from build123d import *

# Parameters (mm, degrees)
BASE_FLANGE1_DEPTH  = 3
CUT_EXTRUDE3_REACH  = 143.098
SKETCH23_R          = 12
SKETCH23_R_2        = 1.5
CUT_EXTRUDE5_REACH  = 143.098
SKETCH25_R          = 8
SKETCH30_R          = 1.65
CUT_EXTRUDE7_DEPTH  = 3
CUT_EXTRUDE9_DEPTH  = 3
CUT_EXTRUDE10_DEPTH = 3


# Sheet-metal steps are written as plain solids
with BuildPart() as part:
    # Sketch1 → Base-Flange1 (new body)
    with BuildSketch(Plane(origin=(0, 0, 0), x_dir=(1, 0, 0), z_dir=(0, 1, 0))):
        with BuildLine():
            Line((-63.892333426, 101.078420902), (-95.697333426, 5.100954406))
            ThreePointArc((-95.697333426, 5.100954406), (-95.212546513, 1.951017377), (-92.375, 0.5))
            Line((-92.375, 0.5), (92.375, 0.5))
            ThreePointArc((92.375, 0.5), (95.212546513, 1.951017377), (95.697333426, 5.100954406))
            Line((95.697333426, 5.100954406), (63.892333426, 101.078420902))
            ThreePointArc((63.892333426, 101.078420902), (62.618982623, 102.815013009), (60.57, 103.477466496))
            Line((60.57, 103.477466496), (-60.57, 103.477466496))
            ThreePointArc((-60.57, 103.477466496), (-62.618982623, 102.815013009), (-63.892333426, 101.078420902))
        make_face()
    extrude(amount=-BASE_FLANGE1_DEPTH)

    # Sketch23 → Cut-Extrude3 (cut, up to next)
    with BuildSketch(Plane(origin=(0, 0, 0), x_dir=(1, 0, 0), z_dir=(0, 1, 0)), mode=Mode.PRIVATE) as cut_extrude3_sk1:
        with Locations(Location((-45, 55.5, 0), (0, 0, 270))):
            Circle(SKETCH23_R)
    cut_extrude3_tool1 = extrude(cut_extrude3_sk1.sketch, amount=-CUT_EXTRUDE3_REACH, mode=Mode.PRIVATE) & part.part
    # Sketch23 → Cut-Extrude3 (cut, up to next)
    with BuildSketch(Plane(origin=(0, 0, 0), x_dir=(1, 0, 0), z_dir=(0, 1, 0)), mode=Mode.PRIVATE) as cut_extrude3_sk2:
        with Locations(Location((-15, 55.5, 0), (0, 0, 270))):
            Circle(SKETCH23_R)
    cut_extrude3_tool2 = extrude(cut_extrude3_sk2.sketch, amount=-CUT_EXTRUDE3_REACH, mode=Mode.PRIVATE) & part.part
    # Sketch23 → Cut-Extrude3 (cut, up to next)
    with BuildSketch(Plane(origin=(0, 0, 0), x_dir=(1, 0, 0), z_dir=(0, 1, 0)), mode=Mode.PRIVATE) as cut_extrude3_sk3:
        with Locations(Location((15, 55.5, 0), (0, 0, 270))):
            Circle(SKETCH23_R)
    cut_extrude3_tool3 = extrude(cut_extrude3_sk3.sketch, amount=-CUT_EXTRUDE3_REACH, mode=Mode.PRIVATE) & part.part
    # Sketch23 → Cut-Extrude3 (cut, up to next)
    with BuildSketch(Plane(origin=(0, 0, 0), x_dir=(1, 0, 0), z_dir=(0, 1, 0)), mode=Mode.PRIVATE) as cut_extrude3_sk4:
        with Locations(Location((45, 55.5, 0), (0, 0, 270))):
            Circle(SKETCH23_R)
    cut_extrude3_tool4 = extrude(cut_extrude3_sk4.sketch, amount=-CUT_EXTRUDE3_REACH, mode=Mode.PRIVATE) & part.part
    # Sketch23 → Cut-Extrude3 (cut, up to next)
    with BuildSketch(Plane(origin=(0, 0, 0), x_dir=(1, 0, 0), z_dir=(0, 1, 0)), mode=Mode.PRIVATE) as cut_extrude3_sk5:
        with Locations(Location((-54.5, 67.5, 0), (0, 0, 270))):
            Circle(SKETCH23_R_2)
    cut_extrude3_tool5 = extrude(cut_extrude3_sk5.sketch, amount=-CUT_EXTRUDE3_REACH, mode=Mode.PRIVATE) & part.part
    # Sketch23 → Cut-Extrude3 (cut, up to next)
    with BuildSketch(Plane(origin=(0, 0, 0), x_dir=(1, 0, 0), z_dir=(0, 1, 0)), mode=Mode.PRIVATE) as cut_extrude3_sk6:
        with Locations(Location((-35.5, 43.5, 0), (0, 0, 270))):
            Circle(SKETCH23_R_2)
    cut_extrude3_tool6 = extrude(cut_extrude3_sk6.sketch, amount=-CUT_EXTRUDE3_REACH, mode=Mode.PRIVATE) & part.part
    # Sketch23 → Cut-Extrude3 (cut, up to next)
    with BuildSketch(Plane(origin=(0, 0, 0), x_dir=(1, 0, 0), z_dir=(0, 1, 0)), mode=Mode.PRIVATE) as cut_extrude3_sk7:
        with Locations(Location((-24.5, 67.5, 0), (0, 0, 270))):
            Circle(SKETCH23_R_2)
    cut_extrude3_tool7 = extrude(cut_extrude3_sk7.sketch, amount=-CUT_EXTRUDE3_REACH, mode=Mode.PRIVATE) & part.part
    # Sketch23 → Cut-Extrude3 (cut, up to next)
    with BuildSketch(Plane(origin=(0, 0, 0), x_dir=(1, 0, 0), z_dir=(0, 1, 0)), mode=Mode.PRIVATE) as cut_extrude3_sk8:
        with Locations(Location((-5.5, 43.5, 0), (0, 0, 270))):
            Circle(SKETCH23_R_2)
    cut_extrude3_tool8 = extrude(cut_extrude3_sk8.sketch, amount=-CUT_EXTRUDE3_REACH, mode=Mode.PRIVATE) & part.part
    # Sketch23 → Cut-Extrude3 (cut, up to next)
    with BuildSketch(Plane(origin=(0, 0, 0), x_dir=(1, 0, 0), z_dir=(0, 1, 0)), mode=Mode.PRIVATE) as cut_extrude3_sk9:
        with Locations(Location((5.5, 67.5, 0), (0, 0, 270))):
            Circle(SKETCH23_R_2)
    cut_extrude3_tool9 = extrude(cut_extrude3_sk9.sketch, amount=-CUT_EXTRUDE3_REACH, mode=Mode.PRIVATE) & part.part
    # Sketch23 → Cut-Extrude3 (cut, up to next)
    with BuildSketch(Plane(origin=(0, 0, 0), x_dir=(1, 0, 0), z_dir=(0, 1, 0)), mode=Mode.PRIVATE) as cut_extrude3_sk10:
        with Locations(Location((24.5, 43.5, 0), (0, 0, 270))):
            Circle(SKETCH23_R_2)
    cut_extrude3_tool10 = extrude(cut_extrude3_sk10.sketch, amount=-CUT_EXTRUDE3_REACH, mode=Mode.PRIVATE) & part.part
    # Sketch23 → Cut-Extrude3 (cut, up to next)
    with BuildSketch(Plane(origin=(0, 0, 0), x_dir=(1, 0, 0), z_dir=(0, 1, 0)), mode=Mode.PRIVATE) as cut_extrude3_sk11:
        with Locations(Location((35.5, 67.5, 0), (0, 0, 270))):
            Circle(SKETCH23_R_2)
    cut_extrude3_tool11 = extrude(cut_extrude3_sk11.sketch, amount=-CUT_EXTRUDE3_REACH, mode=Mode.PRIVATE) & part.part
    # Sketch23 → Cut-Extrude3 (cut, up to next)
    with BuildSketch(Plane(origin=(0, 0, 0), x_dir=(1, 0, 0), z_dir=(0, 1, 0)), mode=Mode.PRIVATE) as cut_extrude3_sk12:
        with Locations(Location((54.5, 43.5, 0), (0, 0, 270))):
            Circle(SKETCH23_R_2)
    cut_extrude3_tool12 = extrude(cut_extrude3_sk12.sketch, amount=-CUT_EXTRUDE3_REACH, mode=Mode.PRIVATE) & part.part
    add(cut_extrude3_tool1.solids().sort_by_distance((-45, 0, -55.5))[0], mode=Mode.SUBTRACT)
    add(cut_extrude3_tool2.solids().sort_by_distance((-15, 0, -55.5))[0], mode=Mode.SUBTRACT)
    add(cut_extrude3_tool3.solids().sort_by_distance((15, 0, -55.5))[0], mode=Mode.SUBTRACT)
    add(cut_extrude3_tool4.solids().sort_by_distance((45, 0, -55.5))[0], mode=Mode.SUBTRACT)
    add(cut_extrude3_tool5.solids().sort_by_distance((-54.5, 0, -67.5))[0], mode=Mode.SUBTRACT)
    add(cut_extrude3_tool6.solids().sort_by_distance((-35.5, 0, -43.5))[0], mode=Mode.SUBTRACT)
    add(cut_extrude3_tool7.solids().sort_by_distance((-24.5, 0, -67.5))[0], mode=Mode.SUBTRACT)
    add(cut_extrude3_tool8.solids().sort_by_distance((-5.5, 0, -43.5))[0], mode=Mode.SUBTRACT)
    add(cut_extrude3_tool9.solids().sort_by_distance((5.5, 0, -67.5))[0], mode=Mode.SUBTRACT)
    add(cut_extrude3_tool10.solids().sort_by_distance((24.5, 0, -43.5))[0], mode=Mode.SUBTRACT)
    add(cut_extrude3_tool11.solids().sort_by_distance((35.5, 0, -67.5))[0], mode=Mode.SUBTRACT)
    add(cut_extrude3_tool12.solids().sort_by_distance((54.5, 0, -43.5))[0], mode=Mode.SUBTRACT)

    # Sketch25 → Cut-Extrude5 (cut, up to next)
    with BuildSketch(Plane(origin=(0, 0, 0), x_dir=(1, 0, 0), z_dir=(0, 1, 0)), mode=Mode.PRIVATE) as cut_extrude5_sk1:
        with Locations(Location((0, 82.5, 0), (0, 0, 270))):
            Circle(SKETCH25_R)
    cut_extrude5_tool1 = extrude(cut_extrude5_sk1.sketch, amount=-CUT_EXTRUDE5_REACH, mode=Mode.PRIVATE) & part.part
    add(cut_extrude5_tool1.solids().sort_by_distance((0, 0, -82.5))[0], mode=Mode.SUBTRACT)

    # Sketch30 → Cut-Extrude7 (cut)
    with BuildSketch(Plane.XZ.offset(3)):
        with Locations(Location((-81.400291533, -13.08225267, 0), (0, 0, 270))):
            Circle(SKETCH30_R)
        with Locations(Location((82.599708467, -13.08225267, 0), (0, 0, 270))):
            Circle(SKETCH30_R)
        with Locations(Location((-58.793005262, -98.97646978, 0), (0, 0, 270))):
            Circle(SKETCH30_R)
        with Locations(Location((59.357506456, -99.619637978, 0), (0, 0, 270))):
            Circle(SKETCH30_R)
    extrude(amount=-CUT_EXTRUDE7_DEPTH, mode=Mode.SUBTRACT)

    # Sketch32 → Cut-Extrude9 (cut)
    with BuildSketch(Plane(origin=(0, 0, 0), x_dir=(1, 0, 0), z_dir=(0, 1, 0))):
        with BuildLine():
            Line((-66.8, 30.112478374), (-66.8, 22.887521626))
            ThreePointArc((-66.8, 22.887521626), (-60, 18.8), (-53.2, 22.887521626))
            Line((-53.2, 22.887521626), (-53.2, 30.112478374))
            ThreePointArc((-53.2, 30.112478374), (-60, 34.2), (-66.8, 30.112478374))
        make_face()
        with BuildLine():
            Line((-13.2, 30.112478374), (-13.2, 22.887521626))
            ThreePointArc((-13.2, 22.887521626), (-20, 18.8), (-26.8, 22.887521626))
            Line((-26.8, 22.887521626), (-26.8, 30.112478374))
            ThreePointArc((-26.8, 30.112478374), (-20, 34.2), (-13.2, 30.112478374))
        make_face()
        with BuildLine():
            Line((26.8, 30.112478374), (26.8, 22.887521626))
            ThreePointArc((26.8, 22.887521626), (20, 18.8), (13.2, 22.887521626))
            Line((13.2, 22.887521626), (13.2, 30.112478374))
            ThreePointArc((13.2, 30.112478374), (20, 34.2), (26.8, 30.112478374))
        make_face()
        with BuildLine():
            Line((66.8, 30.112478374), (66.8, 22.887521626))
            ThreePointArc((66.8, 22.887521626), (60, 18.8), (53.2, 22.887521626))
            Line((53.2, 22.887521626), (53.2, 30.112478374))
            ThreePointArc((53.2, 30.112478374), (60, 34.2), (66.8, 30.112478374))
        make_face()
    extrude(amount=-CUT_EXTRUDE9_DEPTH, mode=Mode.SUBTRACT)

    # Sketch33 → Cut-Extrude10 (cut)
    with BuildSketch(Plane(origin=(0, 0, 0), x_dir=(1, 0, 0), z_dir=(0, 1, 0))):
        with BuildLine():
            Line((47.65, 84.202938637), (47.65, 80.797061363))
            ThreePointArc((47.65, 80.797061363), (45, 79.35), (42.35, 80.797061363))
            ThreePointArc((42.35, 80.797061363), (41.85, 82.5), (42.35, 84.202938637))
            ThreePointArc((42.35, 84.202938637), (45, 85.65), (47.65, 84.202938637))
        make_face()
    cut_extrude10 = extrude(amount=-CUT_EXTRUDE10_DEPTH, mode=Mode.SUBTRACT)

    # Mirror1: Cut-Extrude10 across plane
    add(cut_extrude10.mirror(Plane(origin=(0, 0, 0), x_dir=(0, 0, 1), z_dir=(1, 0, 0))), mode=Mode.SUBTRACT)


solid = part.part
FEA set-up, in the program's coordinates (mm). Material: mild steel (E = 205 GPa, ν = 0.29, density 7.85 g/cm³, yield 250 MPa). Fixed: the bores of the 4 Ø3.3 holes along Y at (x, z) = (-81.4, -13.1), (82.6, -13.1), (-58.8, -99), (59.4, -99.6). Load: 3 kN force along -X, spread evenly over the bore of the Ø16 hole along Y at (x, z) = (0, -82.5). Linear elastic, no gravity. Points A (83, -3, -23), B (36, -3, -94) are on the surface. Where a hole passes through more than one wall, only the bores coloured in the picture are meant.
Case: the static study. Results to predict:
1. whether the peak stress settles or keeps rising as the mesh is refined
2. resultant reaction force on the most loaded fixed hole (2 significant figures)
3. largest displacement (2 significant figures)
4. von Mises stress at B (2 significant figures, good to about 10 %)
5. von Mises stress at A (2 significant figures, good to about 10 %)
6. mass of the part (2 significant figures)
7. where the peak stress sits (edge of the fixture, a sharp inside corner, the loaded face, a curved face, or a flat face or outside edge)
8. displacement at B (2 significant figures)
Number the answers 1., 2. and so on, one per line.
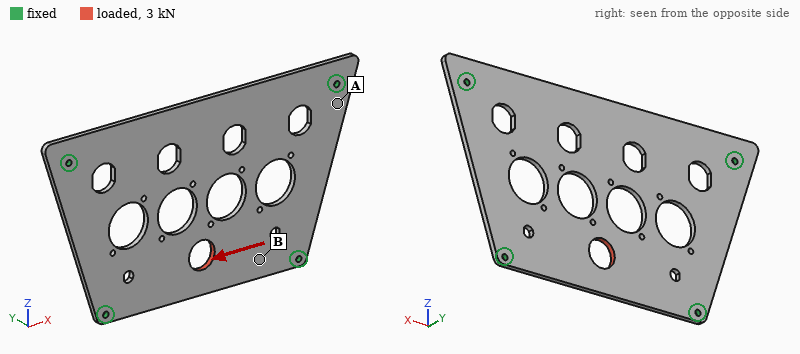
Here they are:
1. keeps rising
2. 1.2 kN
3. 6.5 µm
4. 17 MPa
5. 4.9 MPa
6. 320 g
7. edge of the fixture
8. 3.2 µm
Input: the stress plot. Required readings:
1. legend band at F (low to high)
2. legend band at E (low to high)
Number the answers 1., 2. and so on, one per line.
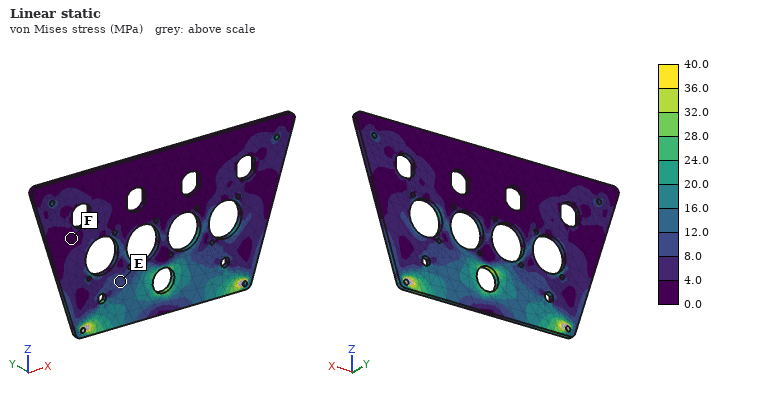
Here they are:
1. 0.0 to 4.0 MPa
2. 8.0 to 12.0 MPa
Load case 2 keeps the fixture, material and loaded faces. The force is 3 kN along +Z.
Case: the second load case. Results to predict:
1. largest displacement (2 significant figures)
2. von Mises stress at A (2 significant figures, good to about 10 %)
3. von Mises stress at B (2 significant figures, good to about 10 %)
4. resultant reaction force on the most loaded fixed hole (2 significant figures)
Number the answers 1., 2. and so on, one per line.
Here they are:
1. 16 µm
2. 12 MPa
3. 13 MPa
4. 1.2 kN
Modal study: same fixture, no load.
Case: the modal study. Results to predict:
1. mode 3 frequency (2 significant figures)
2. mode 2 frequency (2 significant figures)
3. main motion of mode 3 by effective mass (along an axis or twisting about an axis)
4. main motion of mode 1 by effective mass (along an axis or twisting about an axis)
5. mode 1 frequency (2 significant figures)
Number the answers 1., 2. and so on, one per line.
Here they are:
1. 1500 Hz
2. 1100 Hz
3. twisting about Z
4. along Y
5. 580 Hz
